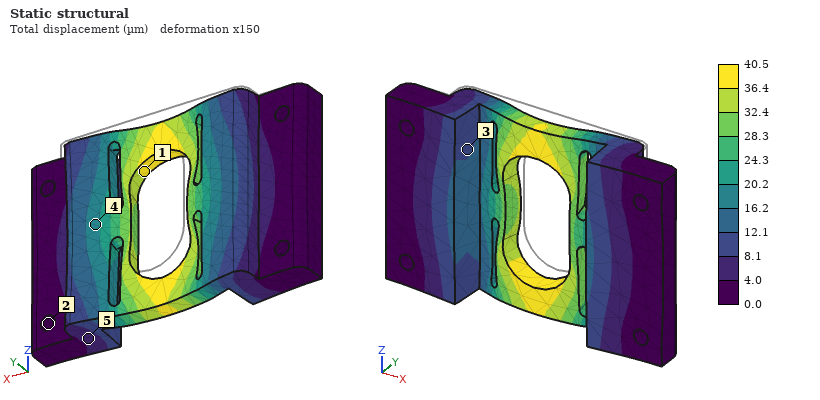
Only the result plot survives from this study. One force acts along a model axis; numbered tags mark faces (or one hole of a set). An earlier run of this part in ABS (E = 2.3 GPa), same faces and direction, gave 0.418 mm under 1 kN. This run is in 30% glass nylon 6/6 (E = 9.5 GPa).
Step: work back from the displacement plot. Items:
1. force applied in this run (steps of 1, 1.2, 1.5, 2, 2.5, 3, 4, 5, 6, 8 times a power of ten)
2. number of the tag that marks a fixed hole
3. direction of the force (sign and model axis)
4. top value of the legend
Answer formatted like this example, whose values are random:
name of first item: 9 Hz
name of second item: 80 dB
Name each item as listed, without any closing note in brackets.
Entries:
force applied in this run: 400 N
number of the tag that marks a fixed hole: 2
direction of the force: -Y
top value of the legend: 40.5 µm
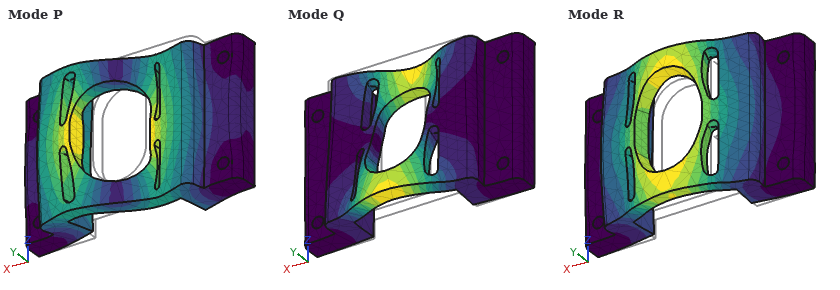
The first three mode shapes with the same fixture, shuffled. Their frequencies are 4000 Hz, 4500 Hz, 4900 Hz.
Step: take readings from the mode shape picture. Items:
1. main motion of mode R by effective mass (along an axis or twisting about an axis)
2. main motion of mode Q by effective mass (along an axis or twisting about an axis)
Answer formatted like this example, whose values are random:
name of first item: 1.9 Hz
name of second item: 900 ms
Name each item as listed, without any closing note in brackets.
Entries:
main motion of mode R by effective mass: along Y
main motion of mode Q by effective mass: twisting about X
